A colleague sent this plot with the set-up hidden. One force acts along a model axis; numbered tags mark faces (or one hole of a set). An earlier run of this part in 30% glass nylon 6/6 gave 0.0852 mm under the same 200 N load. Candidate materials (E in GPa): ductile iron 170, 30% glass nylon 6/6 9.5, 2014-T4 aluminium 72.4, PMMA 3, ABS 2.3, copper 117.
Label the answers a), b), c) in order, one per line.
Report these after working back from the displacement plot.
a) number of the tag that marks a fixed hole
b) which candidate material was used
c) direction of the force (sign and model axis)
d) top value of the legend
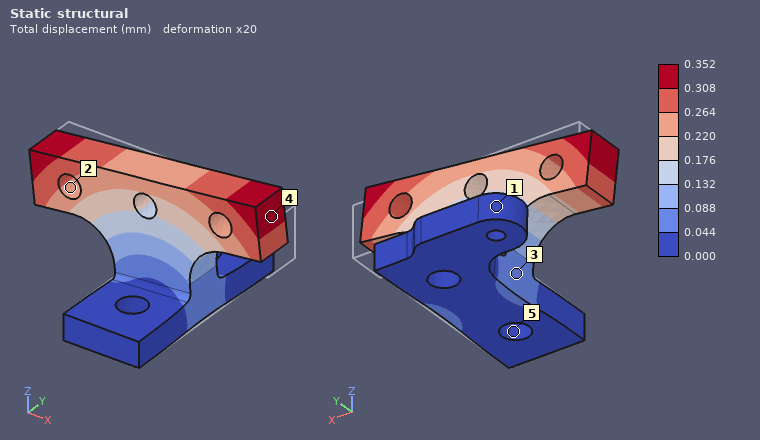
a) 5
b) ABS
c) -X
d) 0.352 mm
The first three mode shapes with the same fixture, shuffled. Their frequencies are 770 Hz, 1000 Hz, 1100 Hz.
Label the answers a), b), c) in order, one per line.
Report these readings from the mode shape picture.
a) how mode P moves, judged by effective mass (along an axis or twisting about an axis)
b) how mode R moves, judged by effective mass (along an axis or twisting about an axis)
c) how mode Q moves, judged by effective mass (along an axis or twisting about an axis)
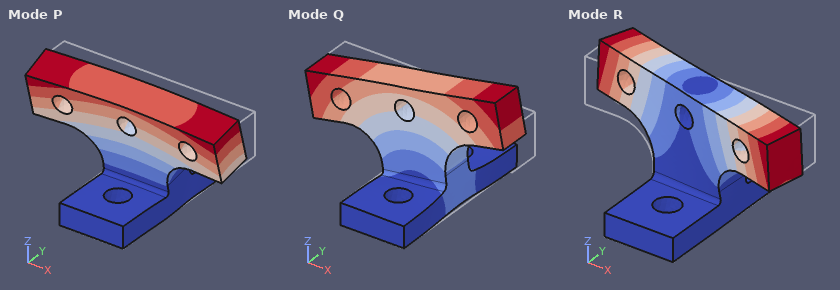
a) along Y
b) twisting about Z
c) along X
